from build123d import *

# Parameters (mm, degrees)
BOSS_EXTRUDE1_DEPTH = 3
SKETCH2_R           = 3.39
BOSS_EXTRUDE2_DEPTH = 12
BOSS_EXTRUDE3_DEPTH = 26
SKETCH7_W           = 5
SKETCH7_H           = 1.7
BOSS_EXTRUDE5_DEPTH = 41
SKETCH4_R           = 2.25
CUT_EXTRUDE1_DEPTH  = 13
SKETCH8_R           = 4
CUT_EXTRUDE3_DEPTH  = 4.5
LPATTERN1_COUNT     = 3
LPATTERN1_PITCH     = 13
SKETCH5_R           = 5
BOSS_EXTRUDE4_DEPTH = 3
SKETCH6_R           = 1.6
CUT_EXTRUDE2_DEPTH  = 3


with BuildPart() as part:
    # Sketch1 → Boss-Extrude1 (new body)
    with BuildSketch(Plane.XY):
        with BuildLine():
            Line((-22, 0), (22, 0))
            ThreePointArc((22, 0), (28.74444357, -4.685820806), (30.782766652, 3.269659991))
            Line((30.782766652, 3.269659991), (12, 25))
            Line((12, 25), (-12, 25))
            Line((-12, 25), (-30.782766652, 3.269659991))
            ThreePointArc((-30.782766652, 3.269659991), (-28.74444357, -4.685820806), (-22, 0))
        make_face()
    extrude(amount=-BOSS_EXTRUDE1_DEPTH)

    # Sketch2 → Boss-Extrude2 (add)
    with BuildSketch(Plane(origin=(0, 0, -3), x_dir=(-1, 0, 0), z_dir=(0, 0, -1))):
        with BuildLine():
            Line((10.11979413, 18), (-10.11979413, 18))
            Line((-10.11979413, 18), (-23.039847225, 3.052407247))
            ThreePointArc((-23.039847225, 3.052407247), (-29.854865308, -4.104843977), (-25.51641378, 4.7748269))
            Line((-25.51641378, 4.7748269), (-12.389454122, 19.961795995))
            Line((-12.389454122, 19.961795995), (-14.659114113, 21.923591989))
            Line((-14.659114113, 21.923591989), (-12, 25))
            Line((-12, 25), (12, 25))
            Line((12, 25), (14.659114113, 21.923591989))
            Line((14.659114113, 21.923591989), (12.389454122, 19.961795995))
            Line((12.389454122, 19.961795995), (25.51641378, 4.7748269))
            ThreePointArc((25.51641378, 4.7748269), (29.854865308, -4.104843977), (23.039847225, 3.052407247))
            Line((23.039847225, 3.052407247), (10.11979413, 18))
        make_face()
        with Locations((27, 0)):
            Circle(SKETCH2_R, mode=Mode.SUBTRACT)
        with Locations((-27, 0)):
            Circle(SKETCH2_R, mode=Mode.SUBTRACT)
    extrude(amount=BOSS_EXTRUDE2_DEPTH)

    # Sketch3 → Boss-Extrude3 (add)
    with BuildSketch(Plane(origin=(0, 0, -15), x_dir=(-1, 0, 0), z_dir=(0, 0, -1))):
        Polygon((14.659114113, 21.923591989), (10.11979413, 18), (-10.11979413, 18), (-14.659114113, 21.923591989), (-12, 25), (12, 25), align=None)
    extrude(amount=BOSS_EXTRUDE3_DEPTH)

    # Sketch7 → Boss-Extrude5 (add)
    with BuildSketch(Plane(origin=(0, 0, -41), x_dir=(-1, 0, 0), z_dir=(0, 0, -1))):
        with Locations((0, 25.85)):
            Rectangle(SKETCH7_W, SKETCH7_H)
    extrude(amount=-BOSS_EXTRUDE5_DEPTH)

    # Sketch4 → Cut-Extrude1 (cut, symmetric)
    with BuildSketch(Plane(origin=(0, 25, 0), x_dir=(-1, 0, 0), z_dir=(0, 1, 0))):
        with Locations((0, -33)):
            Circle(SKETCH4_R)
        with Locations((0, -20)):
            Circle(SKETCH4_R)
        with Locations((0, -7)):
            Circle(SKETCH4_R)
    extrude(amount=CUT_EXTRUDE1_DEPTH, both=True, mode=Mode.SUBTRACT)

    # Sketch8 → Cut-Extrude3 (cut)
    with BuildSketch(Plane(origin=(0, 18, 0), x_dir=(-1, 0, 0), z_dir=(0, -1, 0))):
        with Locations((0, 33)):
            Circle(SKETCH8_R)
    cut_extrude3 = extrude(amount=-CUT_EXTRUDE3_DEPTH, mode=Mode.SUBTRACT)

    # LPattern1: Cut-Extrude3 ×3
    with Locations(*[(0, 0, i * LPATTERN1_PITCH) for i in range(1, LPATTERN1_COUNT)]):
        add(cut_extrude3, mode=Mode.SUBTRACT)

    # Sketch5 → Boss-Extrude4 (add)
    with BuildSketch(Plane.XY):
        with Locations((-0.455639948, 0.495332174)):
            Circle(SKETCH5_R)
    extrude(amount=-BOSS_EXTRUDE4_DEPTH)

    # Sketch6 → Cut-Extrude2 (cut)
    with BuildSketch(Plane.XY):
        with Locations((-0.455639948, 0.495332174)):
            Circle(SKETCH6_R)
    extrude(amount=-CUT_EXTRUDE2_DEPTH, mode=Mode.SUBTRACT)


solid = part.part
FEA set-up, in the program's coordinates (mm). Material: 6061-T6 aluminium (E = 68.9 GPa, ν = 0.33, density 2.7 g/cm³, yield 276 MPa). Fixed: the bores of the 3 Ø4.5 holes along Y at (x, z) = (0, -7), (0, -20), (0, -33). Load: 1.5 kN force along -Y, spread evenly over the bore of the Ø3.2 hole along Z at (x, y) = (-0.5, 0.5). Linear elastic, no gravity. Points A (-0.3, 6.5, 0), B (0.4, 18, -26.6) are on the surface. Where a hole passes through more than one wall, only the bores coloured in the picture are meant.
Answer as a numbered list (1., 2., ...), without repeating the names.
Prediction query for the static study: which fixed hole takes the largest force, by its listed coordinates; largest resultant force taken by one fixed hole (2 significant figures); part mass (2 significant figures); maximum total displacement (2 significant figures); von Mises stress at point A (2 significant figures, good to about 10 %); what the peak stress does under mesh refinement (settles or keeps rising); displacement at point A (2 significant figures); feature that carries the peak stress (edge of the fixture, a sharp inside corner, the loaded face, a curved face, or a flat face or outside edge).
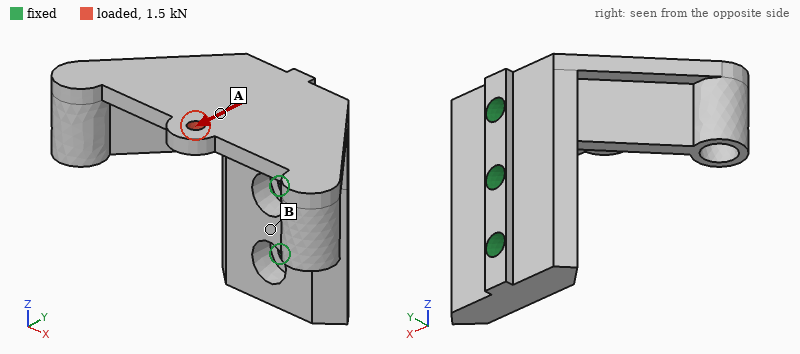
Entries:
1. (0, -7)
2. 1.7 kN
3. 34 g
4. 35 µm
5. 45 MPa
6. keeps rising
7. 24 µm
8. edge of the fixture
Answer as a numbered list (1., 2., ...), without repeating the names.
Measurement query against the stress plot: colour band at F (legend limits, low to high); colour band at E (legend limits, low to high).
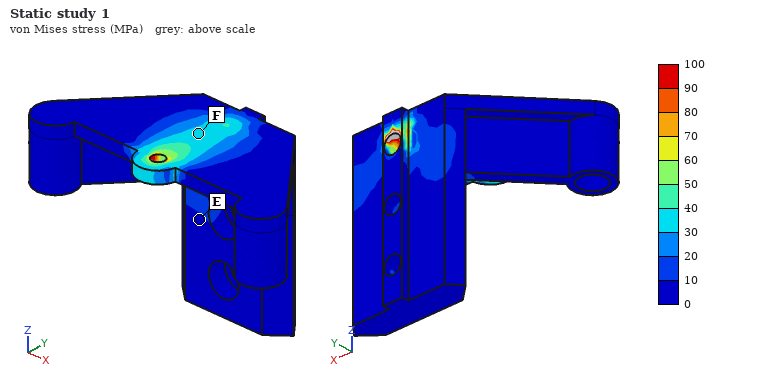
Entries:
1. 30 to 40 MPa
2. 0 to 10 MPa
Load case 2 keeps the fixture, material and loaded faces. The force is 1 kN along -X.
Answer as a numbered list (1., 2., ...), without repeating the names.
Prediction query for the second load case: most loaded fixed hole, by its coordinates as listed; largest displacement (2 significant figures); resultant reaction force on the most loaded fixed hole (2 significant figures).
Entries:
1. (0, -7)
2. 0.27 mm
3. 920 N
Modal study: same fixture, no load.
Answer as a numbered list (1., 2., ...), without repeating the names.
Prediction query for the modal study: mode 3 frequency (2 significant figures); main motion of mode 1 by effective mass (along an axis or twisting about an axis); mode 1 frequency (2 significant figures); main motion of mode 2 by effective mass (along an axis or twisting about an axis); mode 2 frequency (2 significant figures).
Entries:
1. 7000 Hz
2. along X
3. 2900 Hz
4. along Z
5. 5800 Hz
